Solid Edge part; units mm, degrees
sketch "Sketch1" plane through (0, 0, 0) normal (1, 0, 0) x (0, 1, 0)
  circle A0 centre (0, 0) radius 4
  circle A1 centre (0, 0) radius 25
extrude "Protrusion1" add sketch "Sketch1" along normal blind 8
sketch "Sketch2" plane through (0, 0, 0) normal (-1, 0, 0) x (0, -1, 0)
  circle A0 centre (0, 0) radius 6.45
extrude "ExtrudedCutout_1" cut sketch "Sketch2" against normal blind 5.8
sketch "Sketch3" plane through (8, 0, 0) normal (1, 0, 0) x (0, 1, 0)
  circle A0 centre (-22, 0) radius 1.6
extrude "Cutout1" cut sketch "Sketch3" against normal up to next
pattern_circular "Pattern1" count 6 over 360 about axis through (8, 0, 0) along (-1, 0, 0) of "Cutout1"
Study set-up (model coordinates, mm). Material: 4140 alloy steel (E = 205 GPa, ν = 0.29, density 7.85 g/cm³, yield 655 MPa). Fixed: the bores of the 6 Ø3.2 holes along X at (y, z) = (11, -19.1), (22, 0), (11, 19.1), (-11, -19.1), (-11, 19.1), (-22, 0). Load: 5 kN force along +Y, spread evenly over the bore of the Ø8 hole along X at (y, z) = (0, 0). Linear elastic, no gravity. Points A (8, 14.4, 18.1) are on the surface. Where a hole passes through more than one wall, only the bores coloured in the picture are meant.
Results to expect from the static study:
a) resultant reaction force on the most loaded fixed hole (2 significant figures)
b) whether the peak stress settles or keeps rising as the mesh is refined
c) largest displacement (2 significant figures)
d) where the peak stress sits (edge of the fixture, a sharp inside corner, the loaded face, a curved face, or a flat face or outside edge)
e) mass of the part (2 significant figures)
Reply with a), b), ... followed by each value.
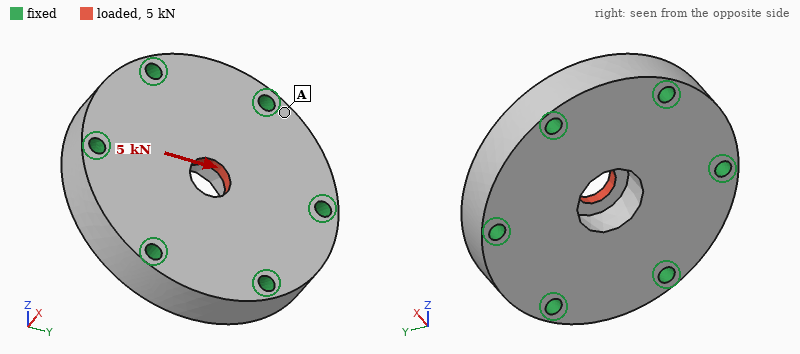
a) 1.3 kN
b) keeps rising
c) 4.0 µm
d) a sharp inside corner
e) 110 g
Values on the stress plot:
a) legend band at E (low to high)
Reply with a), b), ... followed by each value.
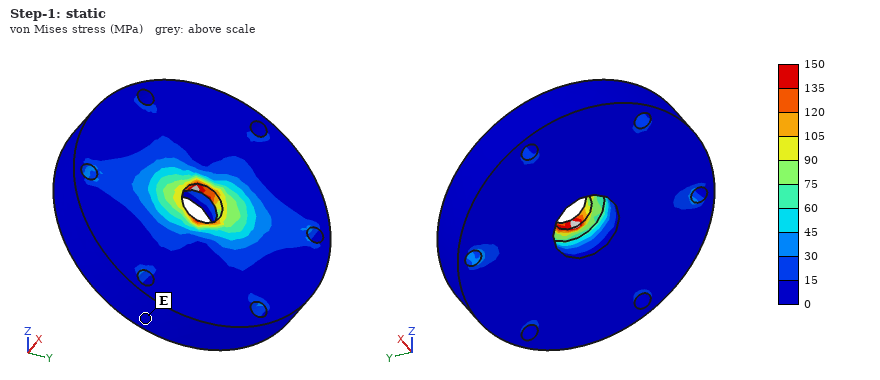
a) 0 to 15 MPa
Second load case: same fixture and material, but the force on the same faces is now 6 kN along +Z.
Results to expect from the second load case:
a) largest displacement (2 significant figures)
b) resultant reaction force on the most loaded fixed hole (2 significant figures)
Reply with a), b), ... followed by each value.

a) 4.8 µm
b) 1.4 kN
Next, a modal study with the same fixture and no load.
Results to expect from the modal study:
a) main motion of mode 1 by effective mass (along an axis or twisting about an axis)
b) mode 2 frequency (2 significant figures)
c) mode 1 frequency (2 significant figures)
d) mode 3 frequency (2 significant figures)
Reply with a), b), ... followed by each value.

a) along X
b) 43 kHz
c) 28 kHz
d) 43 kHz
